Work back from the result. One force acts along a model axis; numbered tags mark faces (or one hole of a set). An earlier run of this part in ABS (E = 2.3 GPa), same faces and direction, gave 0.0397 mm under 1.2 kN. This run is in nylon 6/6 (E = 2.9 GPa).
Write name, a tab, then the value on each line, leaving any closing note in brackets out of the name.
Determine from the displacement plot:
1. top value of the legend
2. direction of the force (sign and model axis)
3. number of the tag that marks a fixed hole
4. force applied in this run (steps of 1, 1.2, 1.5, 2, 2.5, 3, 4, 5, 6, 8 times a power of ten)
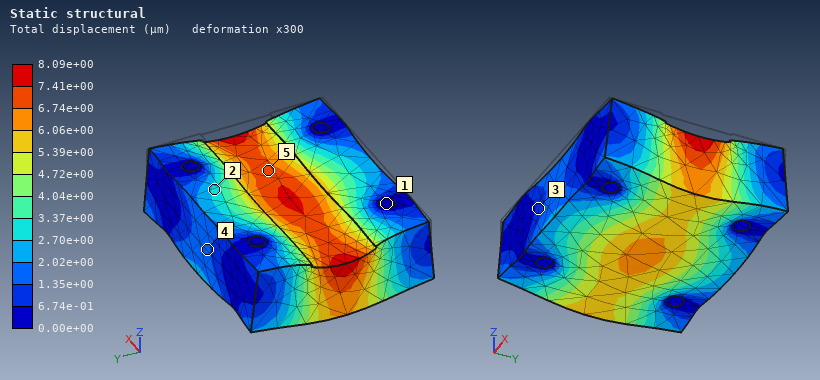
top value of the legend	8.09e+00 µm
direction of the force	-Z
number of the tag that marks a fixed hole	1
force applied in this run	300 N
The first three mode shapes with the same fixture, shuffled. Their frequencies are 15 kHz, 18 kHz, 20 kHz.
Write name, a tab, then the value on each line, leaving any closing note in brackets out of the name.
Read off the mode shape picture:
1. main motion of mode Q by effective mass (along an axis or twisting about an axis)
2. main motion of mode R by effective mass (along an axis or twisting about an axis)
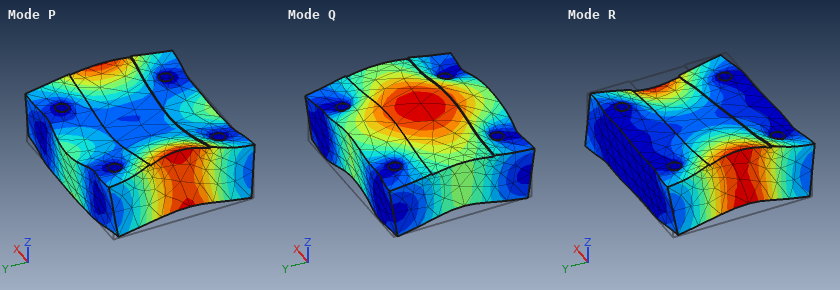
main motion of mode Q by effective mass	along Z
main motion of mode R by effective mass	twisting about Y
